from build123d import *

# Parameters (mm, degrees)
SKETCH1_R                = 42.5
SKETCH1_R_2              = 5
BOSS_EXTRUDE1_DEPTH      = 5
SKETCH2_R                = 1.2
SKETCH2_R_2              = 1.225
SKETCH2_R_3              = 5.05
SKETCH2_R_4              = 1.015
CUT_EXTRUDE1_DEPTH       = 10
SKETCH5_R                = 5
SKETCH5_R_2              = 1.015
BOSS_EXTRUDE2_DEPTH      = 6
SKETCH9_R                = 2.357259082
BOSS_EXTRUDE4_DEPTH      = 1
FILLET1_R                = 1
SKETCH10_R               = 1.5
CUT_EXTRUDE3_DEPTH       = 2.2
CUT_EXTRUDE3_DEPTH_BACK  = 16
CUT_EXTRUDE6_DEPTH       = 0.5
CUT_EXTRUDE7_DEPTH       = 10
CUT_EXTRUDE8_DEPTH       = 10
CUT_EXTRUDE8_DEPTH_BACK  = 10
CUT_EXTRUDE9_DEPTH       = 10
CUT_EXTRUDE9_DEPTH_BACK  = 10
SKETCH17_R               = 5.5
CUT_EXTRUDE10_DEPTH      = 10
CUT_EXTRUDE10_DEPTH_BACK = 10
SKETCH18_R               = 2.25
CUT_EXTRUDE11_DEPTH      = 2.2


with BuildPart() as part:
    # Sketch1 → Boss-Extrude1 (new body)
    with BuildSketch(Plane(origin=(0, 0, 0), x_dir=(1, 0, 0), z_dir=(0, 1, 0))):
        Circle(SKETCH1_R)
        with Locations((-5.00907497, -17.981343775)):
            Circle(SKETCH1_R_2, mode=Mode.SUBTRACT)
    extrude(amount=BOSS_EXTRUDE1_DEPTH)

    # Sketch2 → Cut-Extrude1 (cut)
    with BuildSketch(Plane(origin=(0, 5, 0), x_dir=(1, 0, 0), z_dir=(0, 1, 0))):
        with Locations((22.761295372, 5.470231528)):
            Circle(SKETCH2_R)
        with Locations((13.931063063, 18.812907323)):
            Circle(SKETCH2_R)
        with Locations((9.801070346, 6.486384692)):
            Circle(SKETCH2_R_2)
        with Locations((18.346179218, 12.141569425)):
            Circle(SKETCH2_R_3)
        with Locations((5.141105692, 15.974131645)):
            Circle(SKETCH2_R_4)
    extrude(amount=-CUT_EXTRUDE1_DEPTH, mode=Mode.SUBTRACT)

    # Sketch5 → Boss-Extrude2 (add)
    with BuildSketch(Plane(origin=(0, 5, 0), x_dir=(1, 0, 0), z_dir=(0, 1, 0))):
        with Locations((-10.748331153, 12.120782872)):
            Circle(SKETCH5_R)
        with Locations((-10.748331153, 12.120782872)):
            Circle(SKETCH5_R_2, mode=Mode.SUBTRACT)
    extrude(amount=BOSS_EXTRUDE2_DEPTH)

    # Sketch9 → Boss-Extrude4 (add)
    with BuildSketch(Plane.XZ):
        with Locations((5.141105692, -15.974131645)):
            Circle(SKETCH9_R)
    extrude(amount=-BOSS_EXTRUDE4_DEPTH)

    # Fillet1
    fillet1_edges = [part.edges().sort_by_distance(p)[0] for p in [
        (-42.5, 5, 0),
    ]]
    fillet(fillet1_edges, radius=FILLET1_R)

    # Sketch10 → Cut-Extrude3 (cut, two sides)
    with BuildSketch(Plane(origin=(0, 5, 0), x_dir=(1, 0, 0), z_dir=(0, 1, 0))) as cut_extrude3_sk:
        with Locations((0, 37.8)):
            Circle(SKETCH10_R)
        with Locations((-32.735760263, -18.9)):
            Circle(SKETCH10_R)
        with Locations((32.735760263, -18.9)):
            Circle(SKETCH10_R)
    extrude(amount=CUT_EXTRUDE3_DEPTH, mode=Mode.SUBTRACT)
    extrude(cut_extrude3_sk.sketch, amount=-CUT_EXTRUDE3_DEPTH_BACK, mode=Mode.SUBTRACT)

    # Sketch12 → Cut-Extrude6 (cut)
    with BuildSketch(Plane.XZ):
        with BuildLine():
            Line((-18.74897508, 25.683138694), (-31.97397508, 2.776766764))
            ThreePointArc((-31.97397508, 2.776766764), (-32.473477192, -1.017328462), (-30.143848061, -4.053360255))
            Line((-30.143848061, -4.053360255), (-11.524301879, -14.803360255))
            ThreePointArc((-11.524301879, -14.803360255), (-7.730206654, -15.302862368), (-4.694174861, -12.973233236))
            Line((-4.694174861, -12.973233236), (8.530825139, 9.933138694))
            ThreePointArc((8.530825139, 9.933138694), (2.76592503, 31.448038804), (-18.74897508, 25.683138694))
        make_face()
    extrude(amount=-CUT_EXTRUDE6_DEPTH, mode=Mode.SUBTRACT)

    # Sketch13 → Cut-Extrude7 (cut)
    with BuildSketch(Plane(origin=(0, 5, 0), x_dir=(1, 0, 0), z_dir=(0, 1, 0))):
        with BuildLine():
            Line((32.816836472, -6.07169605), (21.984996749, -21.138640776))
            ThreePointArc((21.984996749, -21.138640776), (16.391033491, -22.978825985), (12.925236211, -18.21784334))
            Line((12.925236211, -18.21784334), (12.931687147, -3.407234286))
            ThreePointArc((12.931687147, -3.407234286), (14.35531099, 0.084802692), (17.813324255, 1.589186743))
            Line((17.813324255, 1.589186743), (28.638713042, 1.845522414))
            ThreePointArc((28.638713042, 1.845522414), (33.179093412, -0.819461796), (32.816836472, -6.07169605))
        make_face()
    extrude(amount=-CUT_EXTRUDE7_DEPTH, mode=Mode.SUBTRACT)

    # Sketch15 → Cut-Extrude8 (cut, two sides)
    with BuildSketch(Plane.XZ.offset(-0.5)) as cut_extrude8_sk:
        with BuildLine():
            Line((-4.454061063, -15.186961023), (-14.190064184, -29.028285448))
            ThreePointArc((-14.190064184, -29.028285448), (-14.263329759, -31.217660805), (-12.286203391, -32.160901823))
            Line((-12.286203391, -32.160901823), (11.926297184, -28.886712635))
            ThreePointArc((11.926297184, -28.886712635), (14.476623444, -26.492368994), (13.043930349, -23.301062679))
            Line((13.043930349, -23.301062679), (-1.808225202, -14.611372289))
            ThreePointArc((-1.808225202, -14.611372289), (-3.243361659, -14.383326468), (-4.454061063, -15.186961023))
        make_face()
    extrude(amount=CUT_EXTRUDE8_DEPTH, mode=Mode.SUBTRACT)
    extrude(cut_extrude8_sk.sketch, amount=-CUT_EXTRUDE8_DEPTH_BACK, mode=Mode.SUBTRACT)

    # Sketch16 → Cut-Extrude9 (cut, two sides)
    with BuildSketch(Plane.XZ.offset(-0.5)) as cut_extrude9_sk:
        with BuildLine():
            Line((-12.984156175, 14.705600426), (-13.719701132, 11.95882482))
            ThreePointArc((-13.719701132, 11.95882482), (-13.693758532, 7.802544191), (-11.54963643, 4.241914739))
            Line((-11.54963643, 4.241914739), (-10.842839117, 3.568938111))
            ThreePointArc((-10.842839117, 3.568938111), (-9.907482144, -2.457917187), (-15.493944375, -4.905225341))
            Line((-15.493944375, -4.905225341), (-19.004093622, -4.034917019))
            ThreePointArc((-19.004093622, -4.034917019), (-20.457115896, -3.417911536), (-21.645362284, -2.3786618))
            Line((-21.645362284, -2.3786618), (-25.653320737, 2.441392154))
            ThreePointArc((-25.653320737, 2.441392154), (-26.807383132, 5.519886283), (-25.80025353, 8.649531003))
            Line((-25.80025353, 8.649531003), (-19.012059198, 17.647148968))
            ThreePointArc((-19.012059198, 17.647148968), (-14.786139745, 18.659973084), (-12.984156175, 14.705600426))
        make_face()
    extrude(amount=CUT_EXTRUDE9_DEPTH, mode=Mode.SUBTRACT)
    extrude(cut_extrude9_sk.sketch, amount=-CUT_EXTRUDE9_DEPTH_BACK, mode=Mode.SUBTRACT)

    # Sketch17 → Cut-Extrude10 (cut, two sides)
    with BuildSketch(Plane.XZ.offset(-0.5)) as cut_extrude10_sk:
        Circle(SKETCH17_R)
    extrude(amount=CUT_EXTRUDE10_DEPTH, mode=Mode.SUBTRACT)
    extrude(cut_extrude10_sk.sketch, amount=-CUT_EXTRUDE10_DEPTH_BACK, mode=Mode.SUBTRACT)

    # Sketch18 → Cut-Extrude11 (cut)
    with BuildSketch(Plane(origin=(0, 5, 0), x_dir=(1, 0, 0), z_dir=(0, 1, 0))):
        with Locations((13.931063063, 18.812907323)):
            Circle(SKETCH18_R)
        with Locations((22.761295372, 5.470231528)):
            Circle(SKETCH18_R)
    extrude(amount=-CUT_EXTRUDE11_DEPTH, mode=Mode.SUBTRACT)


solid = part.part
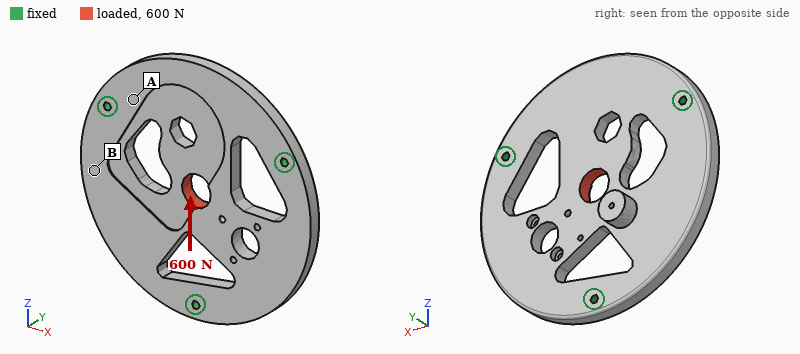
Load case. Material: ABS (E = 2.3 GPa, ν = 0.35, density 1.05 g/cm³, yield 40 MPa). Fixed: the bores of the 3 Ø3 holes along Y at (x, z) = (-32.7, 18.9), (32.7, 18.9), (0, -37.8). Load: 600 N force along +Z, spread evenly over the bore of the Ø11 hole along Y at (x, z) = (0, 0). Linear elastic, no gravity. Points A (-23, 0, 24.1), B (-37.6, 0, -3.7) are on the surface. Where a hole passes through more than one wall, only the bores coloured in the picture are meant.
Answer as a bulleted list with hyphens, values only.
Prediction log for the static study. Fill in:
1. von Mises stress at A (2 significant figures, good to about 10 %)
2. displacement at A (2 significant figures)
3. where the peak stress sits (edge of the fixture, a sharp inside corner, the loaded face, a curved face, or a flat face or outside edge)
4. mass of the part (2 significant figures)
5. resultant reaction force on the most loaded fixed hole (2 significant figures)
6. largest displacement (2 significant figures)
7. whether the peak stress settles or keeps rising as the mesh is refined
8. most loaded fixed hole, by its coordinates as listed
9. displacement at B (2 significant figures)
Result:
- 2.6 MPa
- 0.034 mm
- a sharp inside corner
- 23 g
- 300 N
- 0.14 mm
- keeps rising
- (-32.7, 18.9)
- 0.022 mm
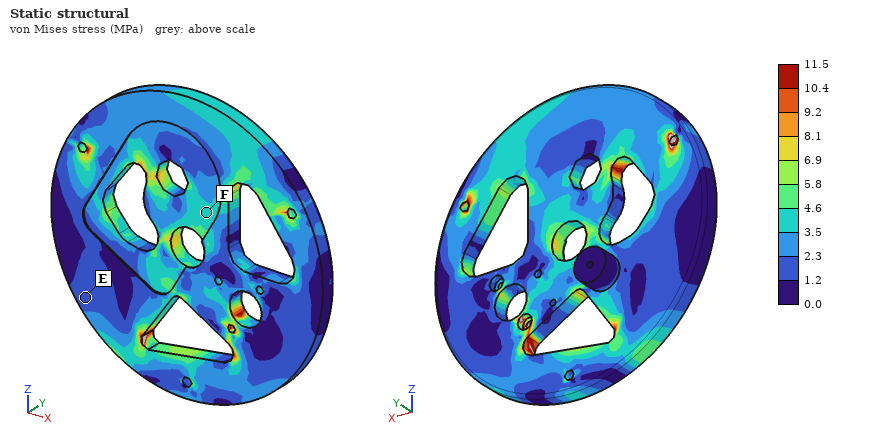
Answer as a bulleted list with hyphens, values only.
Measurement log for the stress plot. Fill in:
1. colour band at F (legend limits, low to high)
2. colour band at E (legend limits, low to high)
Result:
- 3.5 to 4.6 MPa
- 1.2 to 2.3 MPa
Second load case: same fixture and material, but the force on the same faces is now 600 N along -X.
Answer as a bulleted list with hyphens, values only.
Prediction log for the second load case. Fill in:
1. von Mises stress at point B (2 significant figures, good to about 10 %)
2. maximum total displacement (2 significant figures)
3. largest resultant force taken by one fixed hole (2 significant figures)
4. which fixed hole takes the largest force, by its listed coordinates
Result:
- 2.4 MPa
- 0.15 mm
- 260 N
- (0, -37.8)
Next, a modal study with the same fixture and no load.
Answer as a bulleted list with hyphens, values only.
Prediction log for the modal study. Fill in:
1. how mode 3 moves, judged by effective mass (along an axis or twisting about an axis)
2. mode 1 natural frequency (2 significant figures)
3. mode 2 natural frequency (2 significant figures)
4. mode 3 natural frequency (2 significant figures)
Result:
- along Y
- 1000 Hz
- 1100 Hz
- 1100 Hz
